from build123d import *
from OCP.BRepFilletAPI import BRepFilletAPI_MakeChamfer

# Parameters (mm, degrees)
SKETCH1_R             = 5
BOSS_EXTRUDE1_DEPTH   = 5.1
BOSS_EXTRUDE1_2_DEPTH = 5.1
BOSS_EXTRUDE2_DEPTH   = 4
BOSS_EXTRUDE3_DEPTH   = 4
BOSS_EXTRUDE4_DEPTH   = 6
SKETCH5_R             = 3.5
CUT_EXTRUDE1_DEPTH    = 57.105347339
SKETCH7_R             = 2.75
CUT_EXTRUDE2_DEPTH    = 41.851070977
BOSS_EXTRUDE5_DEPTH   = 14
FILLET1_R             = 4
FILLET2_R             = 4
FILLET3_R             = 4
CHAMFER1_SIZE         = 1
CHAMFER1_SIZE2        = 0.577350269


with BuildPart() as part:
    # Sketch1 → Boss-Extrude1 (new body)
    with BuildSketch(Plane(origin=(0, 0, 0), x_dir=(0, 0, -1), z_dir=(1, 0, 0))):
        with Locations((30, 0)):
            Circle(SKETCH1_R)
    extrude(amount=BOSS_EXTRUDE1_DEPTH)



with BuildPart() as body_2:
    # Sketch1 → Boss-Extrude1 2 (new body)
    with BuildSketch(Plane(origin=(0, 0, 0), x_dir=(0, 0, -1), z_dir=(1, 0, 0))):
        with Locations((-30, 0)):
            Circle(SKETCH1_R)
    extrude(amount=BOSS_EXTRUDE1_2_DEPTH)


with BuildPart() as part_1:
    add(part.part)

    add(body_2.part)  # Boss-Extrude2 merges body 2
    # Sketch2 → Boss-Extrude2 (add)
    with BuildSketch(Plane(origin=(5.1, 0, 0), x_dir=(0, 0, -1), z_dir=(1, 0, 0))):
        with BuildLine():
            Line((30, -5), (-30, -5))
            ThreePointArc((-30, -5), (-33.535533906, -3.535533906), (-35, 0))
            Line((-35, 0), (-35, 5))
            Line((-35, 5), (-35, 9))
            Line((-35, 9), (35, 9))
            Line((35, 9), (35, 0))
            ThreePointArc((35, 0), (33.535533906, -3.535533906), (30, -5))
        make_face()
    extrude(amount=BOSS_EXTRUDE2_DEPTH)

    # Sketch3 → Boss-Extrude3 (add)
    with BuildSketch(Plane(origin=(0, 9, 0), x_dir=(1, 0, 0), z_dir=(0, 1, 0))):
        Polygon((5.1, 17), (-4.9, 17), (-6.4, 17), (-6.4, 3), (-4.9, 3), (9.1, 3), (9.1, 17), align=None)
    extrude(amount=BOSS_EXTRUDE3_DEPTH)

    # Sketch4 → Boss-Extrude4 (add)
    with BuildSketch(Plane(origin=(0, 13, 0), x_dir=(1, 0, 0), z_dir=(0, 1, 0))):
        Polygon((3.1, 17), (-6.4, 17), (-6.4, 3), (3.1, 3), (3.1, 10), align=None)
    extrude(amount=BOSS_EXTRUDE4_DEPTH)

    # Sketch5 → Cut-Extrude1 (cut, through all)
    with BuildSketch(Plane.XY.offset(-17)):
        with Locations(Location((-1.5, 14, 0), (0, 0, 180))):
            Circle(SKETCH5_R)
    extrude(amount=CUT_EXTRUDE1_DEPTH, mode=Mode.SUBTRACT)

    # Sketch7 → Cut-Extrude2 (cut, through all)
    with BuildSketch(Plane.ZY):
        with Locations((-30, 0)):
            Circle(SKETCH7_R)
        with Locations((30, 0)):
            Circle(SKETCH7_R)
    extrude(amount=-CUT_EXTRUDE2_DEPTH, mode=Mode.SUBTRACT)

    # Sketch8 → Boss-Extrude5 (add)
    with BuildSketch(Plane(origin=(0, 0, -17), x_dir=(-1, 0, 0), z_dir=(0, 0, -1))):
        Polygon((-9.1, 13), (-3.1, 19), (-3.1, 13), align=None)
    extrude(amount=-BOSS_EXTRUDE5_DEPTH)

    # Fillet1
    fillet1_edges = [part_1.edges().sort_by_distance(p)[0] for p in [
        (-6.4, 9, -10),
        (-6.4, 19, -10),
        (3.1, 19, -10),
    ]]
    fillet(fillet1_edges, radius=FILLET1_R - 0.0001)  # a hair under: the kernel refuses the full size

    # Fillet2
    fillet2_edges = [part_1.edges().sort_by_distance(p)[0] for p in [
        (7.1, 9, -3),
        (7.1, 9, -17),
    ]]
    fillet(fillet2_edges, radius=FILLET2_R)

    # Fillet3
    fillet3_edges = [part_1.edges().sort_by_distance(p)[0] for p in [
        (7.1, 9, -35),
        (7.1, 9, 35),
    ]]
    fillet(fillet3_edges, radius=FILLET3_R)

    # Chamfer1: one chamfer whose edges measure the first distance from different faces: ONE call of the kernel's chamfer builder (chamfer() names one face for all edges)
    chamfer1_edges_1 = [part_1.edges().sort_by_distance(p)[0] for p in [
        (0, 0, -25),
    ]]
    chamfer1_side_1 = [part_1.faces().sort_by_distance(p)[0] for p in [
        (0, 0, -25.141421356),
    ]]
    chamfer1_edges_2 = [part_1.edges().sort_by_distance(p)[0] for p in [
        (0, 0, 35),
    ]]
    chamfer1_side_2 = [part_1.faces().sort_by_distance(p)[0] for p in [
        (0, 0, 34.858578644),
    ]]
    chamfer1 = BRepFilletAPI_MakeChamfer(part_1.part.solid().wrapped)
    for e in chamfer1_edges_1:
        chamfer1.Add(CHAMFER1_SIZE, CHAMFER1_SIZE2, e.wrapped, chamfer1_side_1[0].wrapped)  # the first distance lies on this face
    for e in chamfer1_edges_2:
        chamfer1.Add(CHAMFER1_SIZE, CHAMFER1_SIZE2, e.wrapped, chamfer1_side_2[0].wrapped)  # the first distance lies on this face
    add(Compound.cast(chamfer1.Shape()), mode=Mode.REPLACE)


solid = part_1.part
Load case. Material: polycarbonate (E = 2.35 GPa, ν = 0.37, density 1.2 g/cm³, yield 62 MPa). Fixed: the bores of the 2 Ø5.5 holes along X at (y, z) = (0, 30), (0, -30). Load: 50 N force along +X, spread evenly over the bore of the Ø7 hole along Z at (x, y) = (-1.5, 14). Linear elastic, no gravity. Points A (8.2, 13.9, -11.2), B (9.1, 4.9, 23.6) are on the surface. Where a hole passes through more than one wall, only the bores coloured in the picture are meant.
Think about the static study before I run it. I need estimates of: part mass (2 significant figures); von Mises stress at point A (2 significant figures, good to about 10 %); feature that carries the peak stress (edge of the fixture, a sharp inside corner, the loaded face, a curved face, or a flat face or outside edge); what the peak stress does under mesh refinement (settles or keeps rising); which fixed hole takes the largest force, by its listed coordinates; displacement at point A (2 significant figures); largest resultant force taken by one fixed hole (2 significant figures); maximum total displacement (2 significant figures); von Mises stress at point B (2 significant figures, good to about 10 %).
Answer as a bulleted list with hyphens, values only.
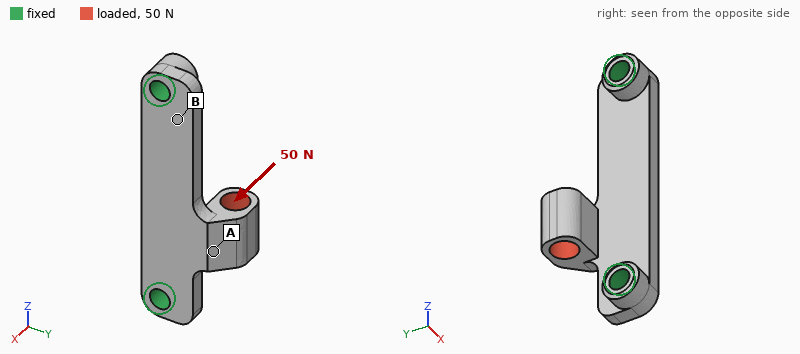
- 6.6 g
- 2.2 MPa
- edge of the fixture
- keeps rising
- (0, -30)
- 0.45 mm
- 37 N
- 0.77 mm
- 5.4 MPa
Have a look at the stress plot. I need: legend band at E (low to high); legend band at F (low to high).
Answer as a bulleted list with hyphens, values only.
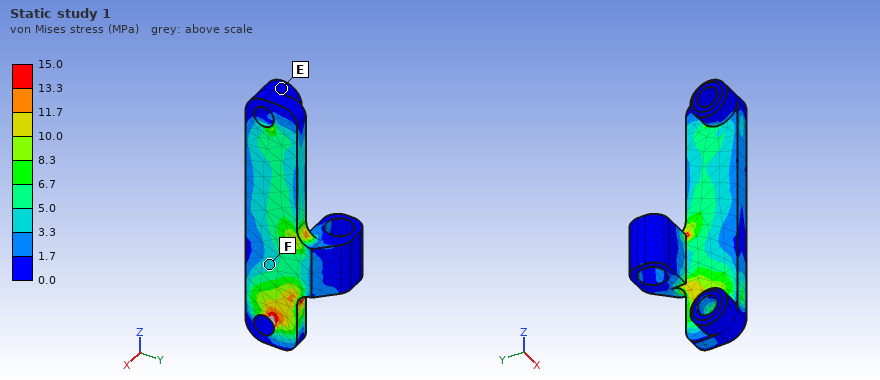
- 0.0 to 1.7 MPa
- 3.3 to 5.0 MPa
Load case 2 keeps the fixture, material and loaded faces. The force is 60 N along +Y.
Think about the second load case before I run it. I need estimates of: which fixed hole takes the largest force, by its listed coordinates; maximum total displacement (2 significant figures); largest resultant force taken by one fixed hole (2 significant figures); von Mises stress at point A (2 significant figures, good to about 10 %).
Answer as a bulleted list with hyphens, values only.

- (0, -30)
- 0.68 mm
- 45 N
- 3.4 MPa
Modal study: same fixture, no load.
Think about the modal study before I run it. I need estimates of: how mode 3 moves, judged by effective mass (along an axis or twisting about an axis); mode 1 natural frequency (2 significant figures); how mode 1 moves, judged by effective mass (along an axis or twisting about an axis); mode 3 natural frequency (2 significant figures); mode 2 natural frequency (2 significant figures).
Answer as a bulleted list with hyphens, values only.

- along Y
- 1100 Hz
- along X
- 3300 Hz
- 1900 Hz
